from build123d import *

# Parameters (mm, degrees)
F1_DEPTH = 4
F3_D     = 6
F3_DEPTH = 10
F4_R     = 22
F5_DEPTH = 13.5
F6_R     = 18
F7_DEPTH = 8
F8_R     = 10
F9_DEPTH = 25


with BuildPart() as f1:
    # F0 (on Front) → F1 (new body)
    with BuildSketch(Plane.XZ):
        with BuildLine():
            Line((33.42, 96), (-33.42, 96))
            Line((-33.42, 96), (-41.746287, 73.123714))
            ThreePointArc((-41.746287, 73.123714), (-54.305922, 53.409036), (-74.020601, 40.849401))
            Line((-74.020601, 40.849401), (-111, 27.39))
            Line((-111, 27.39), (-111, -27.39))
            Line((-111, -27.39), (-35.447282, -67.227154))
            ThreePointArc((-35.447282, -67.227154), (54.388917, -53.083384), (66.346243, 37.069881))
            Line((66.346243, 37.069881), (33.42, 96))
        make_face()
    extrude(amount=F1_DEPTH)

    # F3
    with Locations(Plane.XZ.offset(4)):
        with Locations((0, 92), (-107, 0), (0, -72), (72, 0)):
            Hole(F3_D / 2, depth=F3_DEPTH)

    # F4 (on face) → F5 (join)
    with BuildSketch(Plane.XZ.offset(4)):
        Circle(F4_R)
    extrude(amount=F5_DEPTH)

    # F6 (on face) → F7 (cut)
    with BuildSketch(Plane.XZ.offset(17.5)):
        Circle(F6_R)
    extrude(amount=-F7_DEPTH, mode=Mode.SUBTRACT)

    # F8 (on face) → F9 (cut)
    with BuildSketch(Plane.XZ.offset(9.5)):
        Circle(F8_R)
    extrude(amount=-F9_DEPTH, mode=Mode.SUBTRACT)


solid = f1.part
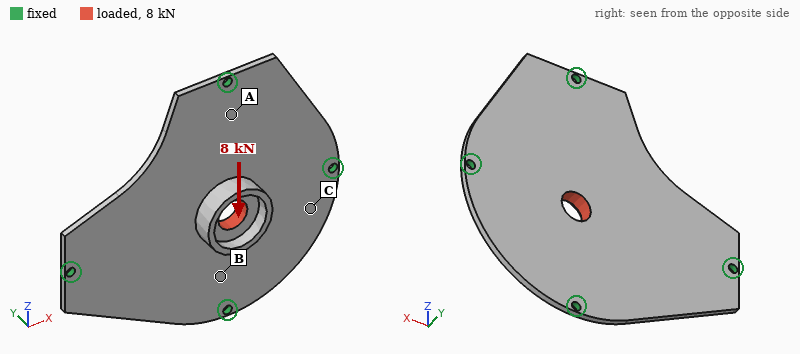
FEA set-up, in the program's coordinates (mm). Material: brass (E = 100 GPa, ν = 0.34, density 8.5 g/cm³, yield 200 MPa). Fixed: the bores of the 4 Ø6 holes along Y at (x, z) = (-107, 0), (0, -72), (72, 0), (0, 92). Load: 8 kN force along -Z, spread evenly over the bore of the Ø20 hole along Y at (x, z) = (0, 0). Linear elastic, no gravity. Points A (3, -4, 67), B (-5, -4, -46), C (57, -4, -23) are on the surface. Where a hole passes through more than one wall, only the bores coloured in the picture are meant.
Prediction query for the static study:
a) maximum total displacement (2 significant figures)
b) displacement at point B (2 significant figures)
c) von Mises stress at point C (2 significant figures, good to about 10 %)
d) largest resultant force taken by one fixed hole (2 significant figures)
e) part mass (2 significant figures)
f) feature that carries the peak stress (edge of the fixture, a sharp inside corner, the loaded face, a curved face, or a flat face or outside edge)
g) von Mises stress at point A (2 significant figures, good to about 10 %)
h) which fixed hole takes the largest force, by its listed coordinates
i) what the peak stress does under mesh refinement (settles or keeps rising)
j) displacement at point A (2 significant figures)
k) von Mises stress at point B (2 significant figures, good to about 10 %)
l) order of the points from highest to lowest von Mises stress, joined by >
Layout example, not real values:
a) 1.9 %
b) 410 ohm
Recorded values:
a) 77 µm
b) 24 µm
c) 8.5 MPa
d) 3.1 kN
e) 860 g
f) edge of the fixture
g) 22 MPa
h) (0, -72)
i) keeps rising
j) 29 µm
k) 33 MPa
l) B > A > C
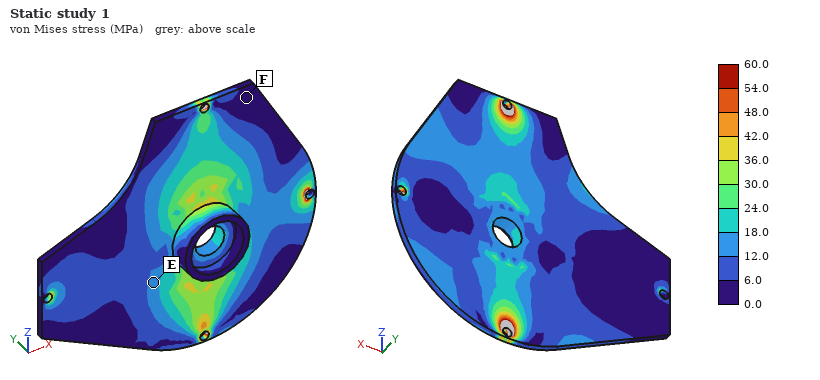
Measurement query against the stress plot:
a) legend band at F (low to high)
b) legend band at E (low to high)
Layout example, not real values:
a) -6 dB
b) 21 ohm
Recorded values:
a) 0.0 to 6.0 MPa
b) 12.0 to 18.0 MPa
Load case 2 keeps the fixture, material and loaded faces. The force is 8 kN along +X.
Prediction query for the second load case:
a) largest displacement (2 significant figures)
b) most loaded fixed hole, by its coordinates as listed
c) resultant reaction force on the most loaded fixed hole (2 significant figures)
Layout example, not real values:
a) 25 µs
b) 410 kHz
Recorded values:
a) 90 µm
b) (72, 0)
c) 3.0 kN
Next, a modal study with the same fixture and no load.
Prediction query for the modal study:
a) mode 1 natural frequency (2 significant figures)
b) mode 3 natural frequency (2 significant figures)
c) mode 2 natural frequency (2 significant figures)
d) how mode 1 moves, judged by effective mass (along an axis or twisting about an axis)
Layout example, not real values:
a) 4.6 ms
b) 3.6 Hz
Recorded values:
a) 570 Hz
b) 970 Hz
c) 920 Hz
d) along Y
